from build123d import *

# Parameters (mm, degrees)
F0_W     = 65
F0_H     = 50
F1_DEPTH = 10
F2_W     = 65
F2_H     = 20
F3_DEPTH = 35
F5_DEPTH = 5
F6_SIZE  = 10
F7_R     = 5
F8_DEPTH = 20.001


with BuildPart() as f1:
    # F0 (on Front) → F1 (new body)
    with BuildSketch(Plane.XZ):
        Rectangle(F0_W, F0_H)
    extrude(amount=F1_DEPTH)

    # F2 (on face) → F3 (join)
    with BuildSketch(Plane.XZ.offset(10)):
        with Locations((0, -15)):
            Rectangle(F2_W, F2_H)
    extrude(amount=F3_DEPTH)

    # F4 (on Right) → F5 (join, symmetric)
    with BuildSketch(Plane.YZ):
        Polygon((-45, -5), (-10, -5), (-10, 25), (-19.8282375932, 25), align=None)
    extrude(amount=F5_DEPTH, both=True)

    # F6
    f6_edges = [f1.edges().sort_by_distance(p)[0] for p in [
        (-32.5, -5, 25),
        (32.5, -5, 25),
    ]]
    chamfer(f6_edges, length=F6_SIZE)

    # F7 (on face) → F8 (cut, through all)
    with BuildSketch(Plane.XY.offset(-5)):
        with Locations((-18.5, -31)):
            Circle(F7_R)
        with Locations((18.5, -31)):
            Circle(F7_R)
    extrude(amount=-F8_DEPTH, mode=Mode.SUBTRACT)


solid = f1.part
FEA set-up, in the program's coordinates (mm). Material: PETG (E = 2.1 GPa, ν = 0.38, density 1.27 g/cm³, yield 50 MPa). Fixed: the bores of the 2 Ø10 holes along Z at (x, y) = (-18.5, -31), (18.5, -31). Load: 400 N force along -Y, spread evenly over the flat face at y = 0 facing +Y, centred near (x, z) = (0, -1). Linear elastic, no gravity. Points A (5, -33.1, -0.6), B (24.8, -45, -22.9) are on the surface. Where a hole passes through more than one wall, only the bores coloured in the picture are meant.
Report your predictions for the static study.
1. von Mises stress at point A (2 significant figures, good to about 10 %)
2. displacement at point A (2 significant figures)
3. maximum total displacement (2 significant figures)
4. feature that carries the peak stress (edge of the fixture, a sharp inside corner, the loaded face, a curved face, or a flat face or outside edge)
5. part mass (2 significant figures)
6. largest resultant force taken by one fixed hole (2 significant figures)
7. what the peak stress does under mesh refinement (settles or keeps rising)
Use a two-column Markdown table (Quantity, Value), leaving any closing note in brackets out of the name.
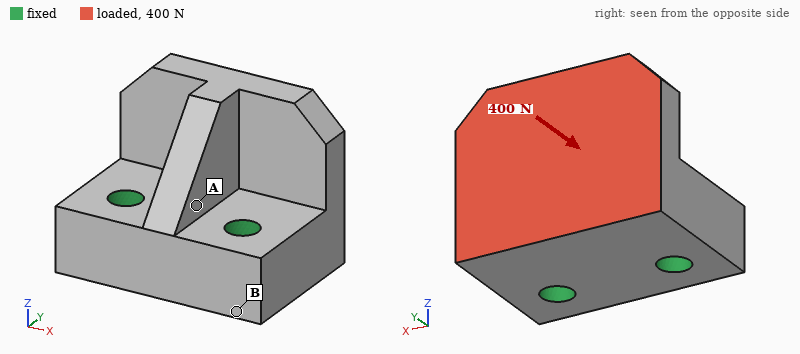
| Quantity | Value |
|---|---|
| von Mises stress at point A | 0.82 MPa |
| displacement at point A | 15 µm |
| maximum total displacement | 76 µm |
| feature that carries the peak stress | edge of the fixture |
| part mass | 100 g |
| largest resultant force taken by one fixed hole | 200 N |
| what the peak stress does under mesh refinement | keeps rising |
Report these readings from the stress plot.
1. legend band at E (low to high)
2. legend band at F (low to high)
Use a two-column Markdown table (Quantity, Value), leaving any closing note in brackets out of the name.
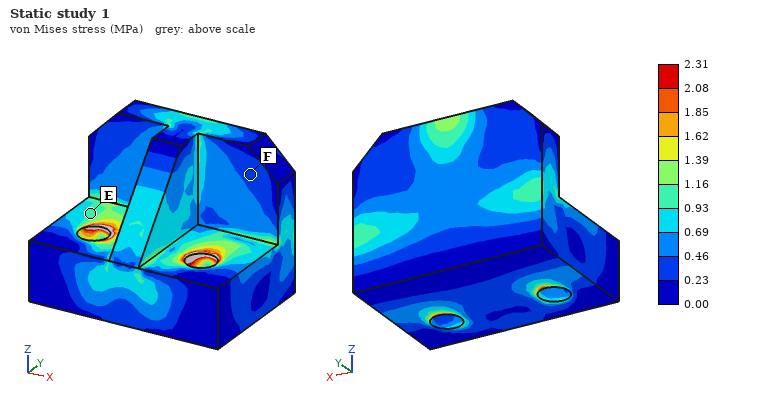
| Quantity | Value |
|---|---|
| legend band at E | 0.93 to 1.16 MPa |
| legend band at F | 0.23 to 0.46 MPa |
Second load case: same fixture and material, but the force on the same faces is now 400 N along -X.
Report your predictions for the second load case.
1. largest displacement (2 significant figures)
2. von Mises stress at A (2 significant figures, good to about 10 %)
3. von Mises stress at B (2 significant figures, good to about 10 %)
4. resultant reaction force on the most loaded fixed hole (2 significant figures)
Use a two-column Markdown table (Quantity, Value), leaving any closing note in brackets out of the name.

| Quantity | Value |
|---|---|
| largest displacement | 52 µm |
| von Mises stress at A | 0.57 MPa |
| von Mises stress at B | 0.23 MPa |
| resultant reaction force on the most loaded fixed hole | 350 N |
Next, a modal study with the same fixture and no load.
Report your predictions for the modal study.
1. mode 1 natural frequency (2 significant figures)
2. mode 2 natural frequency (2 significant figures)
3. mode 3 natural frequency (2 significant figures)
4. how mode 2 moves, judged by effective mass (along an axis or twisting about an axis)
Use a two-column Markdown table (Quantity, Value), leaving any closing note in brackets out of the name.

| Quantity | Value |
|---|---|
| mode 1 natural frequency | 1800 Hz |
| mode 2 natural frequency | 2300 Hz |
| mode 3 natural frequency | 2900 Hz |
| how mode 2 moves, judged by effective mass | along X |
